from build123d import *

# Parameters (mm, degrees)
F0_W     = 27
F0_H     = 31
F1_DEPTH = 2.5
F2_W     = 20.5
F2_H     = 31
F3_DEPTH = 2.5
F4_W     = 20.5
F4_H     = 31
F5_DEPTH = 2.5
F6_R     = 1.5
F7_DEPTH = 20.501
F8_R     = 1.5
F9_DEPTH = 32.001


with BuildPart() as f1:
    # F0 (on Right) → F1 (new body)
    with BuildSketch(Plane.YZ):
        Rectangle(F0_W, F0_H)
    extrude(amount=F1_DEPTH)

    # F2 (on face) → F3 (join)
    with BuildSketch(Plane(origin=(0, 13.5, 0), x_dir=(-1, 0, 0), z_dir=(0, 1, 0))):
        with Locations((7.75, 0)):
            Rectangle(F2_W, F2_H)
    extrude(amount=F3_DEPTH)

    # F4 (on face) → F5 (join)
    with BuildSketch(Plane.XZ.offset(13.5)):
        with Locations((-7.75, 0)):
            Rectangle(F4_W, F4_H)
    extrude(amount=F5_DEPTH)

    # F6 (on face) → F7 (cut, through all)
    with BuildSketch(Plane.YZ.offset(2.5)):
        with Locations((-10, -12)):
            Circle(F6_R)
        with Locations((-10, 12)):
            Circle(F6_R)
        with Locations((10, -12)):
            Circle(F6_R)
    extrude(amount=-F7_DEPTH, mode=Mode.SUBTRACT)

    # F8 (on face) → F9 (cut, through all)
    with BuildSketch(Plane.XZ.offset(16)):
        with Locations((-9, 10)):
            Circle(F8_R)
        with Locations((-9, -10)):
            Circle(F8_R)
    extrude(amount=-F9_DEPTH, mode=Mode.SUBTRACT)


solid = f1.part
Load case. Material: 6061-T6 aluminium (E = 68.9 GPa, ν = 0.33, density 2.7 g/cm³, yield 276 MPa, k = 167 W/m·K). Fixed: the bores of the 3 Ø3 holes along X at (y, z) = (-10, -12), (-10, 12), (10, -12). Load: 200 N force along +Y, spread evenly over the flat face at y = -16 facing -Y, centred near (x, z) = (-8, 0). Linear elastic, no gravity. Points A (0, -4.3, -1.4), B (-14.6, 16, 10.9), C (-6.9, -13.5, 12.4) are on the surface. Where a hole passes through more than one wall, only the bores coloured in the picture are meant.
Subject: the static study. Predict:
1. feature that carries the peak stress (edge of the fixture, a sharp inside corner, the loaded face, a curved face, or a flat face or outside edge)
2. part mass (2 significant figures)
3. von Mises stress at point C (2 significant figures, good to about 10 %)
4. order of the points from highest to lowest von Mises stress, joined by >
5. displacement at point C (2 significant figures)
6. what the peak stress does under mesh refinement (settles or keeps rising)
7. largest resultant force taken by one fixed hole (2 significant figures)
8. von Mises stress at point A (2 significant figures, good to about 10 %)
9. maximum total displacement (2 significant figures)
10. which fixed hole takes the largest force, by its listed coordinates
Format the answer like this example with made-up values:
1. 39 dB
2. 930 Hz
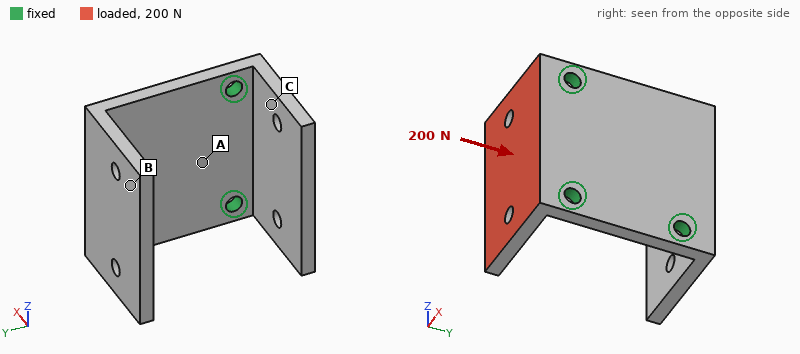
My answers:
1. edge of the fixture
2. 14 g
3. 20 MPa
4. C > A > B
5. 0.035 mm
6. keeps rising
7. 93 N
8. 11 MPa
9. 0.11 mm
10. (-10, 12)
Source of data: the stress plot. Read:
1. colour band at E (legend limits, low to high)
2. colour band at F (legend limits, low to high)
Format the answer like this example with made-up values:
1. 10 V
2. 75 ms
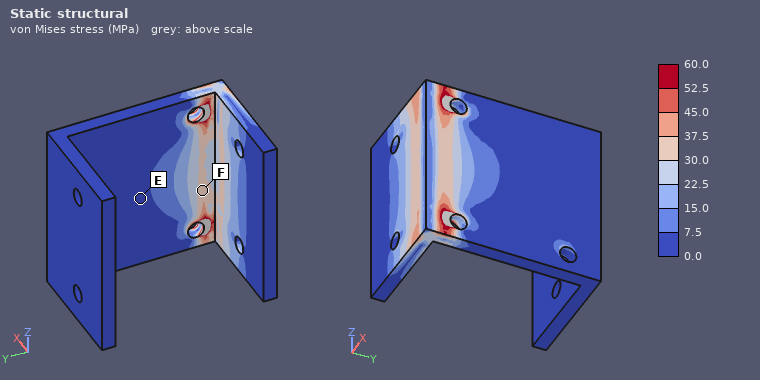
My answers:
1. 0.0 to 7.5 MPa
2. 30.0 to 37.5 MPa
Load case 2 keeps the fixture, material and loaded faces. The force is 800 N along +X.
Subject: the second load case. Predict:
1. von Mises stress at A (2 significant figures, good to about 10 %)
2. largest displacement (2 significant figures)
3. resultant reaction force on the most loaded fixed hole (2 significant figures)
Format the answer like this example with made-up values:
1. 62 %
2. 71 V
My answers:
1. 19 MPa
2. 0.13 mm
3. 430 N
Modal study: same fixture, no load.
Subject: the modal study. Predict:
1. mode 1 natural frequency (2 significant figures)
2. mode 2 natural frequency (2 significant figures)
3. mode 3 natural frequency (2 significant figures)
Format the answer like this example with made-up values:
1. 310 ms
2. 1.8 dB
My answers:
1. 2800 Hz
2. 4100 Hz
3. 4600 Hz
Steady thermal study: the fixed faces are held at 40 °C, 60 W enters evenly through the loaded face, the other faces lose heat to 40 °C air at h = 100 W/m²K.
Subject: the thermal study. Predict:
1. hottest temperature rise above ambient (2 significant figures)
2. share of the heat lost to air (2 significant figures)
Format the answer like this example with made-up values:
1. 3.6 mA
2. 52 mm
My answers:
1. 64 K
2. 9.6 %
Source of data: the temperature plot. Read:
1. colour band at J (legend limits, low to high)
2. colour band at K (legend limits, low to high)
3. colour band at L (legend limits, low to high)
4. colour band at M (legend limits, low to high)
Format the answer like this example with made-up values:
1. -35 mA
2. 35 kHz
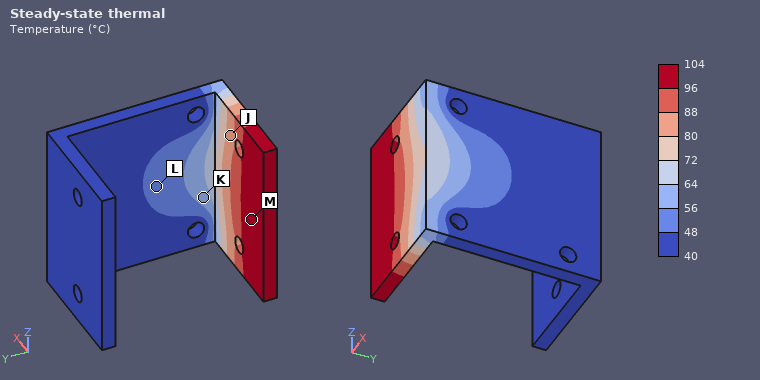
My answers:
1. 80 to 88 °C
2. 56 to 64 °C
3. 48 to 56 °C
4. 96 to 104 °C
